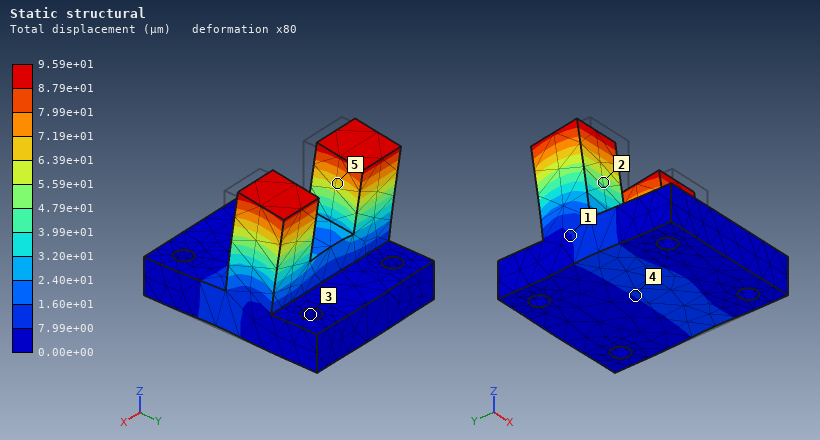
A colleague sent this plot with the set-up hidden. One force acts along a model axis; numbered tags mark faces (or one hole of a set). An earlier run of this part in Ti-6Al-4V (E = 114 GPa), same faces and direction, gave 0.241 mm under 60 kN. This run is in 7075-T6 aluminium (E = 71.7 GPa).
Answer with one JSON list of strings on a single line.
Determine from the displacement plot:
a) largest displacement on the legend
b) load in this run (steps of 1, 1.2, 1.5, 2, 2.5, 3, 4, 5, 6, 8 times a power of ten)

["9.59e+01 µm", "15 kN"]
